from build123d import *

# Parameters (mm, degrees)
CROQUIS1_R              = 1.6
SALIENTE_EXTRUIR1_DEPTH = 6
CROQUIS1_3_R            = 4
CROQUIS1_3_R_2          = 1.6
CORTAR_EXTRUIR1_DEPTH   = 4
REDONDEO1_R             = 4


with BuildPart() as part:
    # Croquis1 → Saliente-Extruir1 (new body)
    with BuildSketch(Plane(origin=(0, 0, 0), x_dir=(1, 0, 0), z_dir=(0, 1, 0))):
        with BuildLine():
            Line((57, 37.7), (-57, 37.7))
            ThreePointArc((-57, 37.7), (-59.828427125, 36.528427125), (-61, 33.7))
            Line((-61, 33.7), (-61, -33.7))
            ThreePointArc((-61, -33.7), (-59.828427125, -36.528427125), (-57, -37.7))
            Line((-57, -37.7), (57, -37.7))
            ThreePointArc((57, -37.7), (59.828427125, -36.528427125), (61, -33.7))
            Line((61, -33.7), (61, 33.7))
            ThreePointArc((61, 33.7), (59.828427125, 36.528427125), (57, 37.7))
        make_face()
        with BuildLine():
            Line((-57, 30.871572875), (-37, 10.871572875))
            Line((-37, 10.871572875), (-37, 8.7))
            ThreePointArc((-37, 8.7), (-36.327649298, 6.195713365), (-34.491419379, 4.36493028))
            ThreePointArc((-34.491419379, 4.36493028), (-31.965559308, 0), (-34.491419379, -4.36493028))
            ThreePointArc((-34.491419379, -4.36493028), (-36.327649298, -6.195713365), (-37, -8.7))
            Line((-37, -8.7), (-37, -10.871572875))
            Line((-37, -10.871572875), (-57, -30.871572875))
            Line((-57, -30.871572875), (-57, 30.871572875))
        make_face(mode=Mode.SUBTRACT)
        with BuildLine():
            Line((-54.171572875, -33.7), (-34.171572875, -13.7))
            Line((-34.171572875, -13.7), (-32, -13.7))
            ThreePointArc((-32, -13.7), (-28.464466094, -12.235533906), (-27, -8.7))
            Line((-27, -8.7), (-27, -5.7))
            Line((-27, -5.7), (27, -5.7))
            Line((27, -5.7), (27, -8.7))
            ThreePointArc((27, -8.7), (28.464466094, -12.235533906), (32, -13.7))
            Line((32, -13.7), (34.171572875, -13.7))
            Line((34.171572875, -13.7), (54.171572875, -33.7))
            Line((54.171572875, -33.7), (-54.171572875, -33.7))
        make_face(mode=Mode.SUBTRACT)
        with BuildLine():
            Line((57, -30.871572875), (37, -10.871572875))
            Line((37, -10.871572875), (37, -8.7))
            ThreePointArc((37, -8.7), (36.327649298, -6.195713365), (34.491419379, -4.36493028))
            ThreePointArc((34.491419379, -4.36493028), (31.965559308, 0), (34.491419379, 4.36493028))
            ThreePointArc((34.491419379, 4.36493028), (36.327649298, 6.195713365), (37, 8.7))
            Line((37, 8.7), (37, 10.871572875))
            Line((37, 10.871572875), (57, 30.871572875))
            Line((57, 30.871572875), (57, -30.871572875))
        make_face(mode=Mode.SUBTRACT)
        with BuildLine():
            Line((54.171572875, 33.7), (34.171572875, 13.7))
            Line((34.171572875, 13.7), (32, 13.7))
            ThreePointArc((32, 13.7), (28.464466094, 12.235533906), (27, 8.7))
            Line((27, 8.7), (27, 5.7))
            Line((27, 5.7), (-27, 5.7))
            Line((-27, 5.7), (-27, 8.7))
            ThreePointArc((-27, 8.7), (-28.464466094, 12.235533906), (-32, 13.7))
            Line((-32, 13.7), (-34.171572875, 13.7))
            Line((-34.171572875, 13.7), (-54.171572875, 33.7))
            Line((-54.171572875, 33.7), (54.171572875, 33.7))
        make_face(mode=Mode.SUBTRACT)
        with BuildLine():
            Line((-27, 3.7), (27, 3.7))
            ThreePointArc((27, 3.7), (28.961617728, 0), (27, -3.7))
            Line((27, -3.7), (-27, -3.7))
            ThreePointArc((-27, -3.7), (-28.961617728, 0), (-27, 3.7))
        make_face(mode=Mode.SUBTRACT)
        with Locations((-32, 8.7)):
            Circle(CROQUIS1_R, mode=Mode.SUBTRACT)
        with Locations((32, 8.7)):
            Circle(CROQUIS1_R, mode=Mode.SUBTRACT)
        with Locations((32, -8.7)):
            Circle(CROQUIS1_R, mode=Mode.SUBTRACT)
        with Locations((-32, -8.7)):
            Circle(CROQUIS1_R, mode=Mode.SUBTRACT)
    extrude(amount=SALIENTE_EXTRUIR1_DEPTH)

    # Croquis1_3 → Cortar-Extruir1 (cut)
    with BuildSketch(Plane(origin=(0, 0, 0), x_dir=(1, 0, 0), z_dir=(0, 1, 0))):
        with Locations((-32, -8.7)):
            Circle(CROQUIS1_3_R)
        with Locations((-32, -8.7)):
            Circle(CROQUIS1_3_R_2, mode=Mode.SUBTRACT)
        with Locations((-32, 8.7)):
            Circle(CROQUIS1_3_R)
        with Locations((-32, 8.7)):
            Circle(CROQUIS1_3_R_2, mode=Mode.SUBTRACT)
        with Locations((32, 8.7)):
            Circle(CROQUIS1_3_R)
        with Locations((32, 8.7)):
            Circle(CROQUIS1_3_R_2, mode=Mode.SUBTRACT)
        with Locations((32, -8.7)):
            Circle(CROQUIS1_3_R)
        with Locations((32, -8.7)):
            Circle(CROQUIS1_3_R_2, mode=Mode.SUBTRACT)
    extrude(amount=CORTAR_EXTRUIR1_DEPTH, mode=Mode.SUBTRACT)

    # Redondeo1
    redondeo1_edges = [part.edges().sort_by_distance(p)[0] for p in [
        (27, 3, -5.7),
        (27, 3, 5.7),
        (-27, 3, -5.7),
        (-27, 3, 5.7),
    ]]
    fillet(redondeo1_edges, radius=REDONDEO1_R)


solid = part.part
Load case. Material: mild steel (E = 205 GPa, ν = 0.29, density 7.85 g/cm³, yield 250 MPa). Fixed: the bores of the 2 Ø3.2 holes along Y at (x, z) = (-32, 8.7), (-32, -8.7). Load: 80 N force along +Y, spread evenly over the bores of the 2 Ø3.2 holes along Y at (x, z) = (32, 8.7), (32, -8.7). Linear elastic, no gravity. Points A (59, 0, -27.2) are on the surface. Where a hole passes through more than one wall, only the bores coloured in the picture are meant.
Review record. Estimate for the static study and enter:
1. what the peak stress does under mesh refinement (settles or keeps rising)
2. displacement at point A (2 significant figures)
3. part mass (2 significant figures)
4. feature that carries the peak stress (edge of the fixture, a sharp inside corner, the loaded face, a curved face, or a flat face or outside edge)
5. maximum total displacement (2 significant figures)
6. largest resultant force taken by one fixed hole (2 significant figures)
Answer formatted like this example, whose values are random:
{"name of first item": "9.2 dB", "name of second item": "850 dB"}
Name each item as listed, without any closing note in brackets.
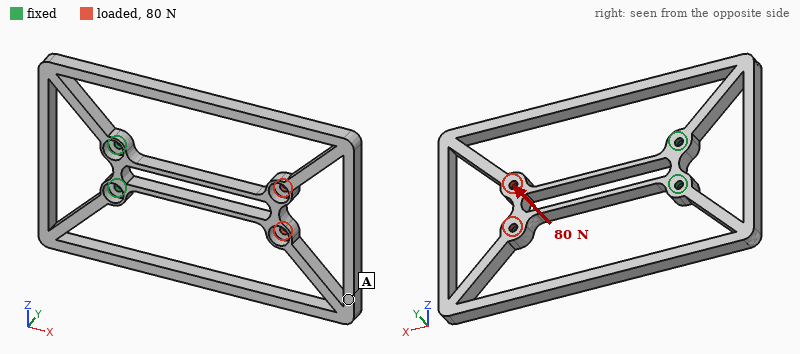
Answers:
{"what the peak stress does under mesh refinement": "keeps rising", "displacement at point A": "0.58 mm", "part mass": "120 g", "feature that carries the peak stress": "edge of the fixture", "maximum total displacement": "0.59 mm", "largest resultant force taken by one fixed hole": "58 N"}
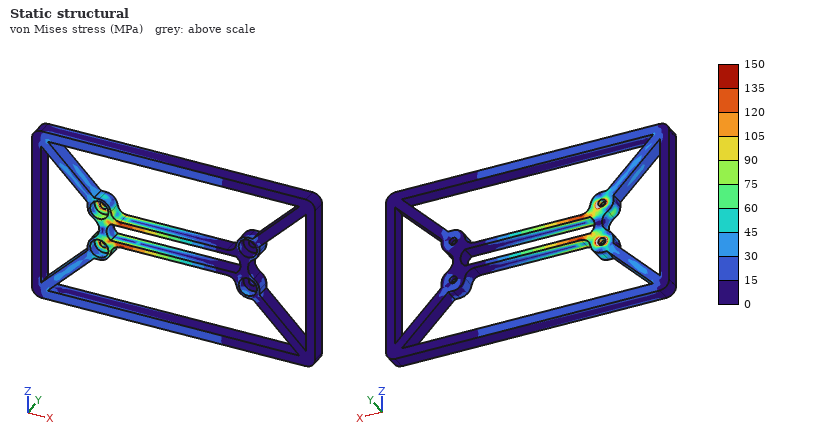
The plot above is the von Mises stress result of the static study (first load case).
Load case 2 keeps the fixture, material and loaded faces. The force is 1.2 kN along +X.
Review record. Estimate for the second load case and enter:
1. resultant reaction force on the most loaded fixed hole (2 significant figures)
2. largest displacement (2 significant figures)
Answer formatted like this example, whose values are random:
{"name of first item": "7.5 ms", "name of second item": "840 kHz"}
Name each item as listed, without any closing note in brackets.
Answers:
{"resultant reaction force on the most loaded fixed hole": "680 N", "largest displacement": "0.34 mm"}
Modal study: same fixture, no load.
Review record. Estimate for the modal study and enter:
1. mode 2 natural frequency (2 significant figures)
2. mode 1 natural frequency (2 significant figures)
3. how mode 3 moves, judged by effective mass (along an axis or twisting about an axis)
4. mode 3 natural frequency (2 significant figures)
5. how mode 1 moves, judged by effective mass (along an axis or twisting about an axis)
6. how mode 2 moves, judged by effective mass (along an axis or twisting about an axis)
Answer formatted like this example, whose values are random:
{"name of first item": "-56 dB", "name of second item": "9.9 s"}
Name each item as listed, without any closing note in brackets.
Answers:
{"mode 2 natural frequency": "300 Hz", "mode 1 natural frequency": "250 Hz", "how mode 3 moves, judged by effective mass": "twisting about X", "mode 3 natural frequency": "460 Hz", "how mode 1 moves, judged by effective mass": "along Y", "how mode 2 moves, judged by effective mass": "along Z"}
